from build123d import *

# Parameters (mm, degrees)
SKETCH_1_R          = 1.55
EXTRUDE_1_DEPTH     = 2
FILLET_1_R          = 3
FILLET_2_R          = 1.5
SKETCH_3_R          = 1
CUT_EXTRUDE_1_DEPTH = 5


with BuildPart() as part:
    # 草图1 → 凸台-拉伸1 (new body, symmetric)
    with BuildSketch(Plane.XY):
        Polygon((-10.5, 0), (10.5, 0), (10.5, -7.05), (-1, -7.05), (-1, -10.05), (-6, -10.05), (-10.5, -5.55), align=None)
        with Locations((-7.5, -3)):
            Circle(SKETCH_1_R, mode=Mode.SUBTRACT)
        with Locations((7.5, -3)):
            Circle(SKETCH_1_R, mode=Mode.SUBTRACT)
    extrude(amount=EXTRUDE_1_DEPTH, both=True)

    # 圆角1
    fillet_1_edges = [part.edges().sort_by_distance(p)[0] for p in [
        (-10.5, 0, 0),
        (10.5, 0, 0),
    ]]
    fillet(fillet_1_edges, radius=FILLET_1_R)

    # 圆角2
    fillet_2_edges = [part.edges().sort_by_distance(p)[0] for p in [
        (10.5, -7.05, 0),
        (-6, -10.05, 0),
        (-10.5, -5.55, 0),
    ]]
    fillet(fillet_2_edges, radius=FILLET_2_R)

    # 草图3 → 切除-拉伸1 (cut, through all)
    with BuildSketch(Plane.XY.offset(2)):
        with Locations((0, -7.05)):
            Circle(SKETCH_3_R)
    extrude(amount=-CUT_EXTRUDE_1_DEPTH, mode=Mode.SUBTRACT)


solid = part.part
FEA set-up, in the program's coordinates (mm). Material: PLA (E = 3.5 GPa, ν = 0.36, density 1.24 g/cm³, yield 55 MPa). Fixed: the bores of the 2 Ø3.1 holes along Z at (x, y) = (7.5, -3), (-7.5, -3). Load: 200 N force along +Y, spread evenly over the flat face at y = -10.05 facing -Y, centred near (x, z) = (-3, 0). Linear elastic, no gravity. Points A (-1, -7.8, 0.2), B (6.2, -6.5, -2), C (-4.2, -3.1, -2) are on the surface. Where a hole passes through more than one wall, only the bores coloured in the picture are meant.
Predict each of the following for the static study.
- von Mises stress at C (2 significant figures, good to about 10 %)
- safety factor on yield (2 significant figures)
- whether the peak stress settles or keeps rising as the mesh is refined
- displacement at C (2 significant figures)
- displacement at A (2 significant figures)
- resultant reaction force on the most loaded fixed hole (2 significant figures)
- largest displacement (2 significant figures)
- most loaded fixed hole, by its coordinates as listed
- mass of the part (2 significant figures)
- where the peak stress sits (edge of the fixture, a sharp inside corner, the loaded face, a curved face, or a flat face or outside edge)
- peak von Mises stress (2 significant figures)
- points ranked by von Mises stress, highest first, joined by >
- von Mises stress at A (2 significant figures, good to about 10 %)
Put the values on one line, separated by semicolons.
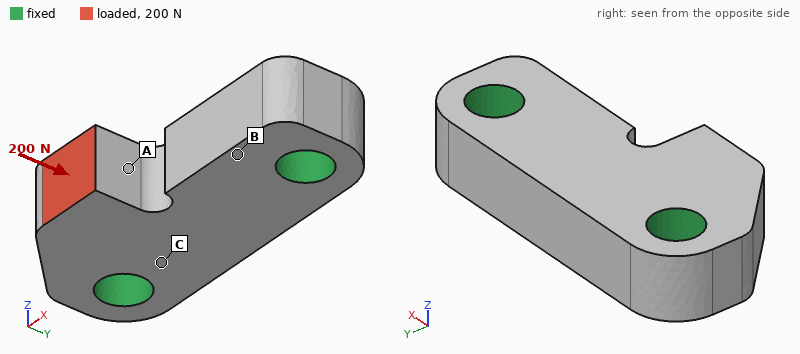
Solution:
8.2 MPa; 1.9; settles; 11 µm; 34 µm; 150 N; 46 µm; (-7.5, -3); 0.72 g; a curved face; 29 MPa; A > C > B; 15 MPa
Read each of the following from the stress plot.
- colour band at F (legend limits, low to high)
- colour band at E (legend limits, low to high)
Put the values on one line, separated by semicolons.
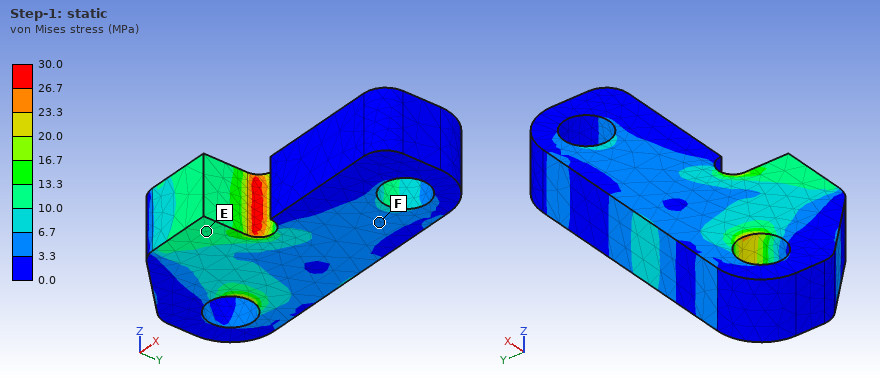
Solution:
3.3 to 6.7 MPa; 10.0 to 13.3 MPa
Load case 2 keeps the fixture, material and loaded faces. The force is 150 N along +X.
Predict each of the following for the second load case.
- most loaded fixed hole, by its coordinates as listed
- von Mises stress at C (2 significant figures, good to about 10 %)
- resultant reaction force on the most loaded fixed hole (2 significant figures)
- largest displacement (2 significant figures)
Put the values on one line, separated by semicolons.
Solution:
(-7.5, -3); 6.4 MPa; 120 N; 73 µm
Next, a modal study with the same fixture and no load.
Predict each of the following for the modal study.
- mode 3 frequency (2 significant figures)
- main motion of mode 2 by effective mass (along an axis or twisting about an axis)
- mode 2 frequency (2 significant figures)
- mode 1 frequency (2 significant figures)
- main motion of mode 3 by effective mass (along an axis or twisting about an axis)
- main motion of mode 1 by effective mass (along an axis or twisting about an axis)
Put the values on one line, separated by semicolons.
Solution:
28 kHz; along Y; 24 kHz; 19 kHz; along Z; along Z
